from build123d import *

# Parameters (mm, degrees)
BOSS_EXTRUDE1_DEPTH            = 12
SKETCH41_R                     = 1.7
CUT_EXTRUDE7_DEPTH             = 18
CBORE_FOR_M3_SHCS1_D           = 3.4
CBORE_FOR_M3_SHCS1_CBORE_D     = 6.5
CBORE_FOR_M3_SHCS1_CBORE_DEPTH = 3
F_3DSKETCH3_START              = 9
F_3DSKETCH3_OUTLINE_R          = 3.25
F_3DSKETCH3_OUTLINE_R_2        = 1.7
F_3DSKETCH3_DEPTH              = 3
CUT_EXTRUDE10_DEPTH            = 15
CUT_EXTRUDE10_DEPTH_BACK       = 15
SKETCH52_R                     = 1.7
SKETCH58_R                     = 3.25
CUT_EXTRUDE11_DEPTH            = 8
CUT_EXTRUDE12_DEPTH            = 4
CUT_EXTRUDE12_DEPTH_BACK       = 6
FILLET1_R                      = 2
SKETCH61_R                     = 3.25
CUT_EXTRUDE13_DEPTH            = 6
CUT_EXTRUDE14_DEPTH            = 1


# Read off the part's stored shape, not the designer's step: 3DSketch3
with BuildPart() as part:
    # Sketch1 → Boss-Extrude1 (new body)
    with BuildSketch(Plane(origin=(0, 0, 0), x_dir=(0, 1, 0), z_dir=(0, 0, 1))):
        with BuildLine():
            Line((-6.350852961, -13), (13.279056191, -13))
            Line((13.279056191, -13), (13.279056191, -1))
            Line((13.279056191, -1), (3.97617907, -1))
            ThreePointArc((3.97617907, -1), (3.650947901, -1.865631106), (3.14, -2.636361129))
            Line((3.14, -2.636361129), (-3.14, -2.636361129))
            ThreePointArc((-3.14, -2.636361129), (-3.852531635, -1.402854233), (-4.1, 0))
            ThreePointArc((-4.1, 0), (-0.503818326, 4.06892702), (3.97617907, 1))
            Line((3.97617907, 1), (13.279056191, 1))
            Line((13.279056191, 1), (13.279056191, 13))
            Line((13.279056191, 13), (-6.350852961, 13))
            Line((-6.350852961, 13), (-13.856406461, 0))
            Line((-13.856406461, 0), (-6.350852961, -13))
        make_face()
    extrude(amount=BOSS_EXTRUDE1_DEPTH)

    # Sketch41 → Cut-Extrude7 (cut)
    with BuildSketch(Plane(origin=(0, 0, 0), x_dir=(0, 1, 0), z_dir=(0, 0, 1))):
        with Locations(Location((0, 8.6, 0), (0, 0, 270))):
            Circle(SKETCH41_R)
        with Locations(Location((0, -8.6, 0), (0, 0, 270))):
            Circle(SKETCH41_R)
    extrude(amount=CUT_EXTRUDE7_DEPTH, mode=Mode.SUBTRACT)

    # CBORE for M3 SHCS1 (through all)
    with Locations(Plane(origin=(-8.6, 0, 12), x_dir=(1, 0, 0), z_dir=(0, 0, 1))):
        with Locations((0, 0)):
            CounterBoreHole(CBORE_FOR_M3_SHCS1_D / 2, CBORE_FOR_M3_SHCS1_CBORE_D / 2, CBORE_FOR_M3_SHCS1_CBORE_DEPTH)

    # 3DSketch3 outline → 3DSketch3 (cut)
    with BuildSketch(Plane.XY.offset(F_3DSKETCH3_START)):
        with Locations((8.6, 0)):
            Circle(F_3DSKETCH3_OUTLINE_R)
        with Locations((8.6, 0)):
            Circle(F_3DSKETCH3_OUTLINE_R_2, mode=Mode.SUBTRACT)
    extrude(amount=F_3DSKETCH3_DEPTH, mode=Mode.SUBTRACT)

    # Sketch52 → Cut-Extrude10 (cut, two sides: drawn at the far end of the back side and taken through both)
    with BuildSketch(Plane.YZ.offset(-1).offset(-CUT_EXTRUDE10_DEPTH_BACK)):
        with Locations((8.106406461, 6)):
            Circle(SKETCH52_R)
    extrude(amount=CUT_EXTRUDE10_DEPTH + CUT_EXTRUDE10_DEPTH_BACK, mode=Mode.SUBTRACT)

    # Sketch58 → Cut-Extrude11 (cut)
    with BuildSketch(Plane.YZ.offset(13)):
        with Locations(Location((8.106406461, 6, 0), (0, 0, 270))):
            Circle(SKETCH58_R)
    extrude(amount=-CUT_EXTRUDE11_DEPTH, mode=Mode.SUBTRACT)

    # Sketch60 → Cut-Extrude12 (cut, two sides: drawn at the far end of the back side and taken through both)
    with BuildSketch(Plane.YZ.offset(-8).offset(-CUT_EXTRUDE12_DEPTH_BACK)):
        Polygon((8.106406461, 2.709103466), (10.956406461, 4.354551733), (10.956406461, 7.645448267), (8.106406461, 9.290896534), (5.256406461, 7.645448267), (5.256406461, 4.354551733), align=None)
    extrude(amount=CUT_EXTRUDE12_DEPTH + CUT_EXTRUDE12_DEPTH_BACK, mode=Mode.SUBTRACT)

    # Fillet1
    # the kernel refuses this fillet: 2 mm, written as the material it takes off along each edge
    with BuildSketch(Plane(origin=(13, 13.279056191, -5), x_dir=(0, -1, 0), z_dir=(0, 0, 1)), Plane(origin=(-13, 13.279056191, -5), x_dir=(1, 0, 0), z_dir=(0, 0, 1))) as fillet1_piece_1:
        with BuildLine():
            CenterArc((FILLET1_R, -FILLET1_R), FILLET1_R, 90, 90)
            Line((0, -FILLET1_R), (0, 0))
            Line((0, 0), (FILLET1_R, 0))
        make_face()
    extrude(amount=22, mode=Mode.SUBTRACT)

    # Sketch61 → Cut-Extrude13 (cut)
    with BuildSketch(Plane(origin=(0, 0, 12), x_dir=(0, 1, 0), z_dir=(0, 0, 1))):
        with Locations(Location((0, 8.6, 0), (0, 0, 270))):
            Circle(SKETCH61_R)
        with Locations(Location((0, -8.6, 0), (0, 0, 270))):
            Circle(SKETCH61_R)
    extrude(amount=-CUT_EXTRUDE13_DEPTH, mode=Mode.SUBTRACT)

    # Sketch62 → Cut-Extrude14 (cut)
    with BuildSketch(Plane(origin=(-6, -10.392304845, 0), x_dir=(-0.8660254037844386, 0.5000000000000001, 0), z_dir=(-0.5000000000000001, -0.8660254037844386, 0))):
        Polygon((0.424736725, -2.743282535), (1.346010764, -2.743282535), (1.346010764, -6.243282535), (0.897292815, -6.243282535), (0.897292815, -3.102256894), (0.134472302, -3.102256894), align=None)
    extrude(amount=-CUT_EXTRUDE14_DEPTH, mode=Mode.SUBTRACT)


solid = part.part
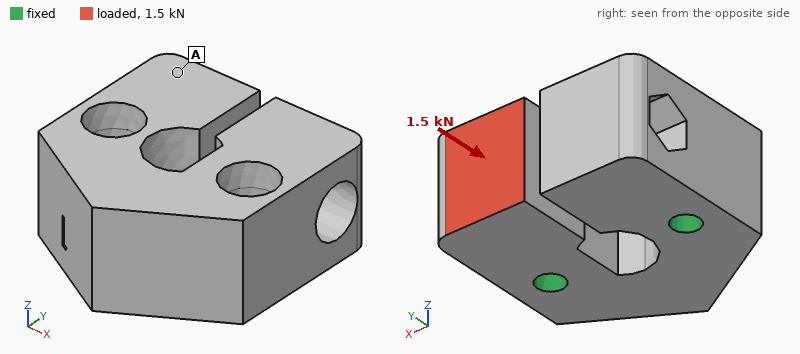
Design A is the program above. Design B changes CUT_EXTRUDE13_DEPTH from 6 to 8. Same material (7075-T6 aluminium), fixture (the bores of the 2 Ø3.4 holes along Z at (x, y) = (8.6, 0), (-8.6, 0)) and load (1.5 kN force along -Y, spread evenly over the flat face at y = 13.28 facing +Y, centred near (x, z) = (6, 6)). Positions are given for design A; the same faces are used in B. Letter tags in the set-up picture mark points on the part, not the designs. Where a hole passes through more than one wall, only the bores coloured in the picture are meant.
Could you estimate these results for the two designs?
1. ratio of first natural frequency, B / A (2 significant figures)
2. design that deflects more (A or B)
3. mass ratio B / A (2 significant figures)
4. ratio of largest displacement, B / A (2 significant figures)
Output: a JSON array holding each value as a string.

["0.67", "B", "0.98", "1.8"]
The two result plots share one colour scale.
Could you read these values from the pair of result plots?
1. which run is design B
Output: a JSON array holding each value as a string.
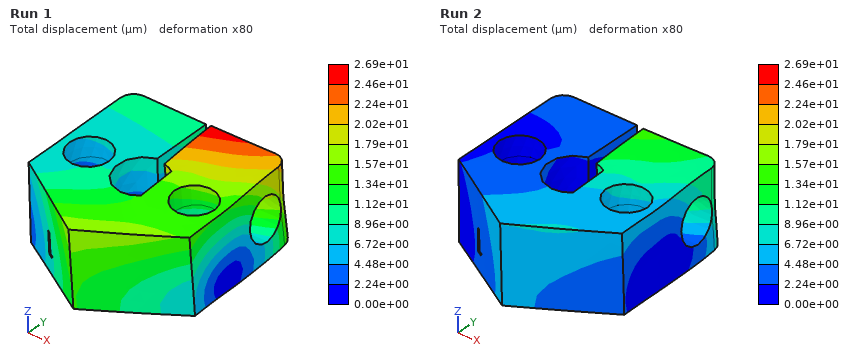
["Run 1"]
